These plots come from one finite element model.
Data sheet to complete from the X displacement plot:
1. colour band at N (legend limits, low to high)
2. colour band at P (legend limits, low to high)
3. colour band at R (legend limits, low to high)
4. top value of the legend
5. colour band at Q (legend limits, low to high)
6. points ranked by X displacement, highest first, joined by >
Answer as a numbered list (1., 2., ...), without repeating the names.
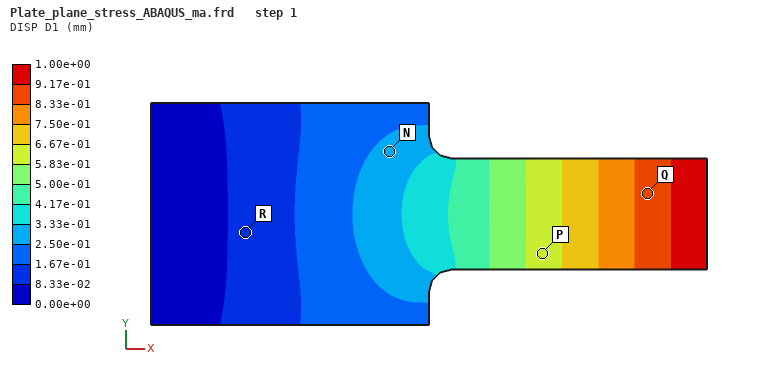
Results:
1. 2.50e-01 to 3.33e-01 mm
2. 5.83e-01 to 6.67e-01 mm
3. 8.33e-02 to 1.67e-01 mm
4. 1.00e+00 mm
5. 8.33e-01 to 9.17e-01 mm
6. Q > P > N > R
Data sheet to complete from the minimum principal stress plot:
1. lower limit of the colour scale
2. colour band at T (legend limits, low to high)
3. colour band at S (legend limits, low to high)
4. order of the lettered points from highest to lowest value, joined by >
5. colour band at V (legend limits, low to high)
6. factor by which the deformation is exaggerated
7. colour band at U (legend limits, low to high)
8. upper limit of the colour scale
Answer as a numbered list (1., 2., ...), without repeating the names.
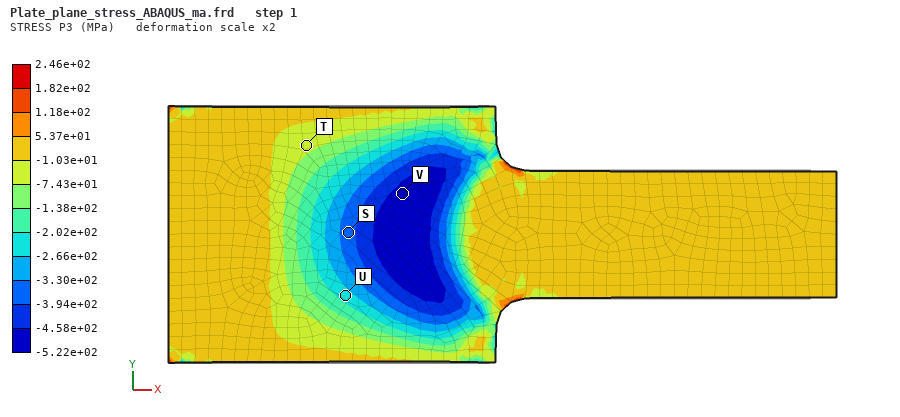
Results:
1. -5.22e+02 MPa
2. -7.43e+01 to -1.03e+01 MPa
3. -3.94e+02 to -3.30e+02 MPa
4. T > U > S > V
5. -5.22e+02 to -4.58e+02 MPa
6. 2
7. -2.66e+02 to -2.02e+02 MPa
8. 2.46e+02 MPa
